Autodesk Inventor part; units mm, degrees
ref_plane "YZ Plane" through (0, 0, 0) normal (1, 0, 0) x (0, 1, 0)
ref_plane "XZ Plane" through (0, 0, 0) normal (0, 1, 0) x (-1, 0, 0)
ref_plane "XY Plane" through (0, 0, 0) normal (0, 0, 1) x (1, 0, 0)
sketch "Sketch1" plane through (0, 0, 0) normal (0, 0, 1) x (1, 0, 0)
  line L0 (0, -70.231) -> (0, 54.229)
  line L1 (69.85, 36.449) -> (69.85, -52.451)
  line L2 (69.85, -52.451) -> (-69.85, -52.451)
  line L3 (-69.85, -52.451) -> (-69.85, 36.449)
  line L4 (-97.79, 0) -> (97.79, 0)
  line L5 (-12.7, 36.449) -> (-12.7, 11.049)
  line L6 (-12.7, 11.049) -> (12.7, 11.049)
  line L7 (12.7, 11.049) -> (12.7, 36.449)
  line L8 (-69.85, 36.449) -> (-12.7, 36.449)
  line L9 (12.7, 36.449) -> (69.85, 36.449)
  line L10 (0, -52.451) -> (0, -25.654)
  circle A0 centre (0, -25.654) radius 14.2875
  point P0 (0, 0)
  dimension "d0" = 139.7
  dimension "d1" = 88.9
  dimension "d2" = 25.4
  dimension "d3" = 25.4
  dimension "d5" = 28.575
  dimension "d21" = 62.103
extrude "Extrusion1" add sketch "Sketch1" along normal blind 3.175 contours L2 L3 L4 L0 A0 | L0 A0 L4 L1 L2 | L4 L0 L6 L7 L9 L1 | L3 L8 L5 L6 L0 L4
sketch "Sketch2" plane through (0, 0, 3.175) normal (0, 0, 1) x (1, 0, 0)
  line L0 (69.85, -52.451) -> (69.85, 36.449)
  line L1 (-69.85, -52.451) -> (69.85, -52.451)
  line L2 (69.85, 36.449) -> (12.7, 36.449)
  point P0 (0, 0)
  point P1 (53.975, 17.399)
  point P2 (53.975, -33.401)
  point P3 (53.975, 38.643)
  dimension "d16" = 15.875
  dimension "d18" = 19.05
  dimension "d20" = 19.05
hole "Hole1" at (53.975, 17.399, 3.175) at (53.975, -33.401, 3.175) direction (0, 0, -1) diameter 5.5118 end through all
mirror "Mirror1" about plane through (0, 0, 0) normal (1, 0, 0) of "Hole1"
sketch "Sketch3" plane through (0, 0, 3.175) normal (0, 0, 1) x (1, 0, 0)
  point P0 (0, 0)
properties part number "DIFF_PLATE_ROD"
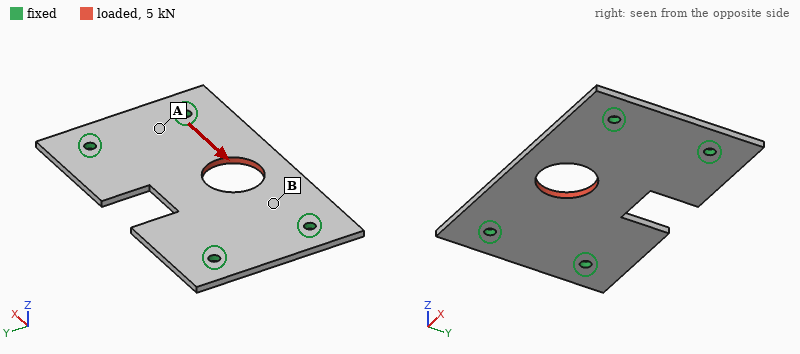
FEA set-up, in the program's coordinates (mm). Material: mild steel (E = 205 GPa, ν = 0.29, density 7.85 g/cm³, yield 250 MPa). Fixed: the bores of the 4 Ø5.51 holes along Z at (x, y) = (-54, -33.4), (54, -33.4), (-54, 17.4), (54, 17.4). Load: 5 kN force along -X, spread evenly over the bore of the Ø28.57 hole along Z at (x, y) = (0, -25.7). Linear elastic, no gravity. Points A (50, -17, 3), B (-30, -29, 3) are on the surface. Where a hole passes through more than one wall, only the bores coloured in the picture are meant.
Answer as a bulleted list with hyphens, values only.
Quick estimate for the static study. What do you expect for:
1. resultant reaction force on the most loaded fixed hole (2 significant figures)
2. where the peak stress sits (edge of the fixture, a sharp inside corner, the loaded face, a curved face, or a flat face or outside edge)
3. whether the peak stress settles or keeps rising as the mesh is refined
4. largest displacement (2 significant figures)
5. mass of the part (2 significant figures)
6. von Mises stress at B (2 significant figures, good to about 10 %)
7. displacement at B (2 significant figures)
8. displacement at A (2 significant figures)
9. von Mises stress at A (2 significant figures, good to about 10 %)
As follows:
- 1.7 kN
- edge of the fixture
- keeps rising
- 5.1 µm
- 280 g
- 19 MPa
- 2.5 µm
- 1.4 µm
- 6.1 MPa
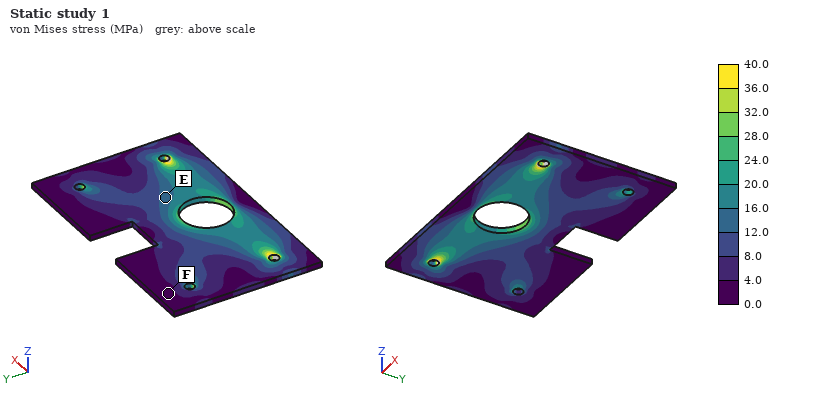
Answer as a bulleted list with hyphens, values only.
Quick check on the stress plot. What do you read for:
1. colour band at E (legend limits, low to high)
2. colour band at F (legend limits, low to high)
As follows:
- 12.0 to 16.0 MPa
- 0.0 to 4.0 MPa
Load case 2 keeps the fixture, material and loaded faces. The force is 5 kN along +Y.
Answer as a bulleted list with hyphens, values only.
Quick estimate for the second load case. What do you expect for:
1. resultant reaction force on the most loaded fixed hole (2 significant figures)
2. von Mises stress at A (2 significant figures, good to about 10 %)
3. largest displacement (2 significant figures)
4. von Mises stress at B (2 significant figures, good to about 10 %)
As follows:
- 1.9 kN
- 17 MPa
- 13 µm
- 23 MPa
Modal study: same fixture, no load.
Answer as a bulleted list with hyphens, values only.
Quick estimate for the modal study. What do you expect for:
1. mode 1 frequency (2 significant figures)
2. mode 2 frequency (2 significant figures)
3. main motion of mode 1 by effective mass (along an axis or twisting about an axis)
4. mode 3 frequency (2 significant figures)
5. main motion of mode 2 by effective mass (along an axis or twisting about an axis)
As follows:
- 1400 Hz
- 1900 Hz
- along Z
- 2800 Hz
- twisting about X
